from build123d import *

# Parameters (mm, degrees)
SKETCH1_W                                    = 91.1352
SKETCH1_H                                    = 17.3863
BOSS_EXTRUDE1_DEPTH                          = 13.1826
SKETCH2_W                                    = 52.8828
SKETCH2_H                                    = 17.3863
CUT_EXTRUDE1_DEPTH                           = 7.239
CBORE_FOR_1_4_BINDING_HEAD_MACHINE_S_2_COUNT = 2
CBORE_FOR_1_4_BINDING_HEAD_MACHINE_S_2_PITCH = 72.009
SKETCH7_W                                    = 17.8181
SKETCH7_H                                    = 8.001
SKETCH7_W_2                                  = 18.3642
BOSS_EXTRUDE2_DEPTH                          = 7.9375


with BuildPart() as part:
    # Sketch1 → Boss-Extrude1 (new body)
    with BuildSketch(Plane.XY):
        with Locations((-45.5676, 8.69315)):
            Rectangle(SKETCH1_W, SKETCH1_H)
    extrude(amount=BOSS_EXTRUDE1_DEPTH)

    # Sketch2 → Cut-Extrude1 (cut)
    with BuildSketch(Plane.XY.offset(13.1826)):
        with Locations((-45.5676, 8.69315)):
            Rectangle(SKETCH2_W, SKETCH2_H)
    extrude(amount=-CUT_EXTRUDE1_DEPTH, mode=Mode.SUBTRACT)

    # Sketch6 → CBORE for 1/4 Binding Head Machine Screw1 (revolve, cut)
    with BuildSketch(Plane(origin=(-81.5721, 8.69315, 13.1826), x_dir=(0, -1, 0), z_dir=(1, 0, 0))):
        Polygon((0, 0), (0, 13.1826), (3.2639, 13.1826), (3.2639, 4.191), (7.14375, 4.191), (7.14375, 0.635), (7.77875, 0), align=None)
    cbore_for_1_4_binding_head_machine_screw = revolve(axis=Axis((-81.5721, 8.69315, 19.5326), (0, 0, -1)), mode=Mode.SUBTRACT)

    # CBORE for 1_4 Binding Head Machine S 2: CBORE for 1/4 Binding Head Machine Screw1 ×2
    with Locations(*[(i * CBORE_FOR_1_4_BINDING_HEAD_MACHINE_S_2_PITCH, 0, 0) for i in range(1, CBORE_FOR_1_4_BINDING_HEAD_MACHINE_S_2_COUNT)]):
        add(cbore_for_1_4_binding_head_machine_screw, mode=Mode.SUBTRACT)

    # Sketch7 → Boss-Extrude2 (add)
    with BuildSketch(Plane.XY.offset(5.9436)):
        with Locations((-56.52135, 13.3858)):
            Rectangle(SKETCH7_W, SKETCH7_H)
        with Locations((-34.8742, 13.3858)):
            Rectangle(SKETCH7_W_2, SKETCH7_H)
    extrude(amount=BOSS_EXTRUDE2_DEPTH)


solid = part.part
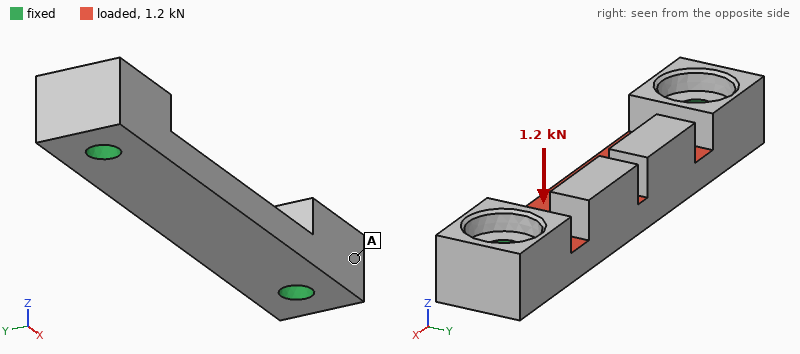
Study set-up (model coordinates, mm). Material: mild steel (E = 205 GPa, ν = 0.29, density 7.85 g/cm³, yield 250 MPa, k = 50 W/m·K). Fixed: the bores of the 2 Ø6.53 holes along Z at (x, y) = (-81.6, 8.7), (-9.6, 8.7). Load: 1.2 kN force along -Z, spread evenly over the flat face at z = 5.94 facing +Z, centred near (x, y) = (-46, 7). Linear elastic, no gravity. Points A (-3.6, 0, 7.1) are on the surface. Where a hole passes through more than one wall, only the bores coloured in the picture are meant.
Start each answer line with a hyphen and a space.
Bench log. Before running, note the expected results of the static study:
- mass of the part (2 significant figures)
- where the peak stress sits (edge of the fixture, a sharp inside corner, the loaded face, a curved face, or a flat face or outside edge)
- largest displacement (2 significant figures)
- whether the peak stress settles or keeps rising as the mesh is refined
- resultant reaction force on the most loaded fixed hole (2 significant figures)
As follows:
- 110 g
- edge of the fixture
- 14 µm
- keeps rising
- 610 N
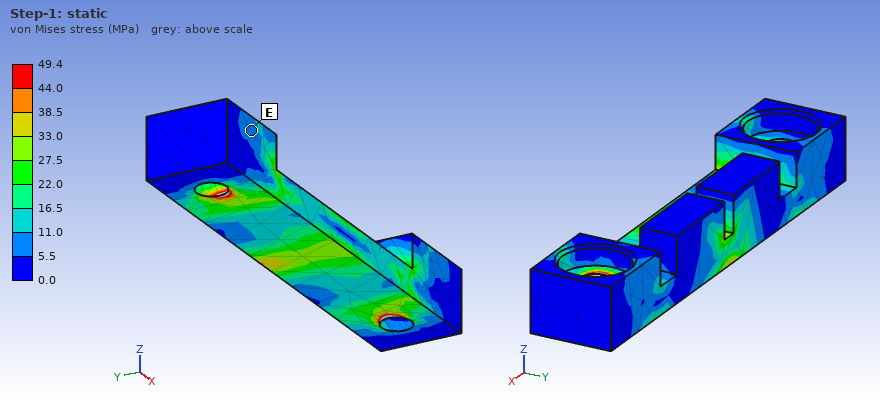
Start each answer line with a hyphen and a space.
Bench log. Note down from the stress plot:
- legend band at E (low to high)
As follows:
- 5.5 to 11.0 MPa
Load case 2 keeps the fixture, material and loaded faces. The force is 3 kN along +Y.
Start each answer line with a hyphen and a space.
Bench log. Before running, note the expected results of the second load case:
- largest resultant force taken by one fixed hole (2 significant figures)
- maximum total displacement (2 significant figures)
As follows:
- 1.5 kN
- 18 µm
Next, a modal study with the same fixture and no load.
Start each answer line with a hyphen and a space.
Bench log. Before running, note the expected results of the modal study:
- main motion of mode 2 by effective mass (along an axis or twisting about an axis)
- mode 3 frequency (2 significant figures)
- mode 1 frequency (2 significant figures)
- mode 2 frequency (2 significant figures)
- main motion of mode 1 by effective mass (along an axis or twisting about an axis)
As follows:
- along Y
- 14 kHz
- 6900 Hz
- 9900 Hz
- along Z
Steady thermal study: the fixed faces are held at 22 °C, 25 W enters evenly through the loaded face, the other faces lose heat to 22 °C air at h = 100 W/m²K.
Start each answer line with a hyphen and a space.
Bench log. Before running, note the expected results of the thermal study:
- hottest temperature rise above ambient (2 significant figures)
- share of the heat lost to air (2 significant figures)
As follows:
- 32 K
- 28 %
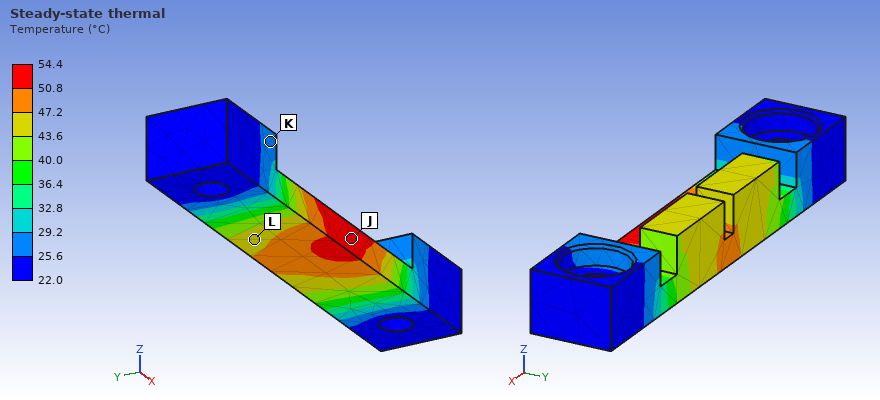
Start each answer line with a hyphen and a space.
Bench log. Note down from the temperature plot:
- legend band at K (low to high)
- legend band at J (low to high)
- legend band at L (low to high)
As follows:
- 25.6 to 29.2 °C
- 50.8 to 54.4 °C
- 43.6 to 47.2 °C
